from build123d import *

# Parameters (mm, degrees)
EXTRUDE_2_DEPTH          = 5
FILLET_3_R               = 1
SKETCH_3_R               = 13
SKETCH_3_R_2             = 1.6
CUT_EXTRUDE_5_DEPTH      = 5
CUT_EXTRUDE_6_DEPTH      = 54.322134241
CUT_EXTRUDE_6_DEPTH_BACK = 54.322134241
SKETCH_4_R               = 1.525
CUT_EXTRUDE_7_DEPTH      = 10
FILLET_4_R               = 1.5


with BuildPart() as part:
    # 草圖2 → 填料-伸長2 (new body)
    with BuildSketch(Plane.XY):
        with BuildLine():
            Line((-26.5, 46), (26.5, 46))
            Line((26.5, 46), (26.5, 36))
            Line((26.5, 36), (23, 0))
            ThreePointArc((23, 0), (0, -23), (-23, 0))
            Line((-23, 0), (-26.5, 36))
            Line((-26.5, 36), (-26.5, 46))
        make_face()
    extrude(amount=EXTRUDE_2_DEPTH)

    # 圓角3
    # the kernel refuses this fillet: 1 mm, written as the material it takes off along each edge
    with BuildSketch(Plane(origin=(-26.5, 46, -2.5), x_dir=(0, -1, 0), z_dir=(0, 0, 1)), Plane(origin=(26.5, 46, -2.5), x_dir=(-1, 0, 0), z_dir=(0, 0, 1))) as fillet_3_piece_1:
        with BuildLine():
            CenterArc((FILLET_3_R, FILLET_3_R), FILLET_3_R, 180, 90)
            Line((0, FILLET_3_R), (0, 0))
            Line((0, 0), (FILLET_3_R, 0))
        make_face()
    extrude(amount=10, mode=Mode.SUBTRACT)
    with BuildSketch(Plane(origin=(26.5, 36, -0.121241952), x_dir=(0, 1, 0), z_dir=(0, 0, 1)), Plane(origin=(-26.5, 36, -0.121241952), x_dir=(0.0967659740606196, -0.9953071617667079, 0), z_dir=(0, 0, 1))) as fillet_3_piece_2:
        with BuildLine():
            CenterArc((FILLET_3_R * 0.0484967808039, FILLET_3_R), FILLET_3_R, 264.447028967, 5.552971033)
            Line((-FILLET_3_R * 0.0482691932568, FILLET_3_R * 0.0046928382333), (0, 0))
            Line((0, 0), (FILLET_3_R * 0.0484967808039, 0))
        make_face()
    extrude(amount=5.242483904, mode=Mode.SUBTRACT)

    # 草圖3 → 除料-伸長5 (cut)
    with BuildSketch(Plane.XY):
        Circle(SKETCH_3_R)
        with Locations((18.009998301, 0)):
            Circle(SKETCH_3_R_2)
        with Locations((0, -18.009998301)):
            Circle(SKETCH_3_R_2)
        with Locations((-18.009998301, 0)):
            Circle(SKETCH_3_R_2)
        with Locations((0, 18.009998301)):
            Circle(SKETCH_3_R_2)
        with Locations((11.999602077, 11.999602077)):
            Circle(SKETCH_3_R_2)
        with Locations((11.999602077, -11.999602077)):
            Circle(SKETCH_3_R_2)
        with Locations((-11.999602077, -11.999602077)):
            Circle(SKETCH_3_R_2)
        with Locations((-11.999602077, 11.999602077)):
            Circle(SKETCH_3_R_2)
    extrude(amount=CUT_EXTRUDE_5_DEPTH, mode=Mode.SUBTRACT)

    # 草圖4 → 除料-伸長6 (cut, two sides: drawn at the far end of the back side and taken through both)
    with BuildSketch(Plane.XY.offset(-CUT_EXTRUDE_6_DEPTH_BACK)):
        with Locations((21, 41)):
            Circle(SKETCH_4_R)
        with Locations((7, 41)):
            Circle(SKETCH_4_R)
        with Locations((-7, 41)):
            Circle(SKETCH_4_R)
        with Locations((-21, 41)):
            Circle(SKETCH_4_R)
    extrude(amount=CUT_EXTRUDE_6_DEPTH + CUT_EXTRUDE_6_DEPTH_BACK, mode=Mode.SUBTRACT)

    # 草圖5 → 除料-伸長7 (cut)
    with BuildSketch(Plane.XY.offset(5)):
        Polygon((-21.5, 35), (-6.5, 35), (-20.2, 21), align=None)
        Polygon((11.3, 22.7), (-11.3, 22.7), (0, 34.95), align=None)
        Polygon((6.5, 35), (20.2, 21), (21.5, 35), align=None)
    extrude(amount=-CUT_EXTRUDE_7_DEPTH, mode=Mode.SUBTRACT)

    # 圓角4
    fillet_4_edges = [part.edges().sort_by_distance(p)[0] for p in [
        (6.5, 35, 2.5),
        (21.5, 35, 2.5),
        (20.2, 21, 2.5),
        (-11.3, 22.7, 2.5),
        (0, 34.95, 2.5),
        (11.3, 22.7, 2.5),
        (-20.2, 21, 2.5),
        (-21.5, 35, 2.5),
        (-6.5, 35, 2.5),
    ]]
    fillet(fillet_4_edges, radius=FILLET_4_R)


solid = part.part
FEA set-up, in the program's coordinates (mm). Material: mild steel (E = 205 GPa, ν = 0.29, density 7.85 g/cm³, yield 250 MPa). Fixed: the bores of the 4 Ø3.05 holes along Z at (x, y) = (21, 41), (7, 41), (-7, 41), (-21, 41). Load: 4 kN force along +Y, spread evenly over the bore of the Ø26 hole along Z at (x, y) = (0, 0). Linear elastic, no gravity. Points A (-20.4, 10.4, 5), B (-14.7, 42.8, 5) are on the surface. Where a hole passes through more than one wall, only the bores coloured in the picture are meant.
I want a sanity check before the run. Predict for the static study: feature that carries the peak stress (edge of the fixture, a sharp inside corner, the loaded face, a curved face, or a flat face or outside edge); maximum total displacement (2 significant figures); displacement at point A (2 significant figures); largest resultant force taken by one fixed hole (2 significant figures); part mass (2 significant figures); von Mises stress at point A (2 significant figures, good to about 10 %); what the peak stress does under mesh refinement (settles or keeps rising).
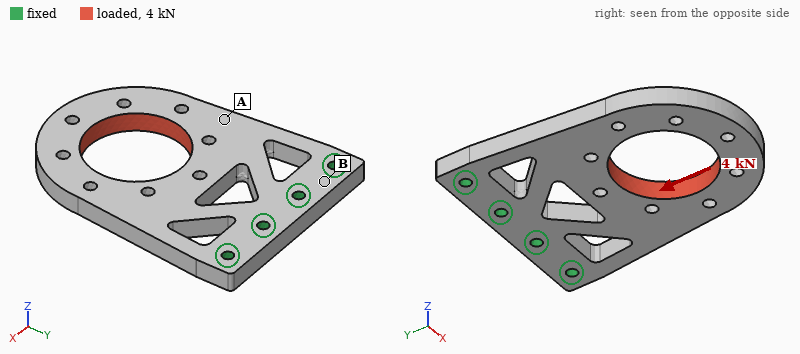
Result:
a sharp inside corner
12 µm
6.2 µm
1.1 kN
86 g
27 MPa
keeps rising
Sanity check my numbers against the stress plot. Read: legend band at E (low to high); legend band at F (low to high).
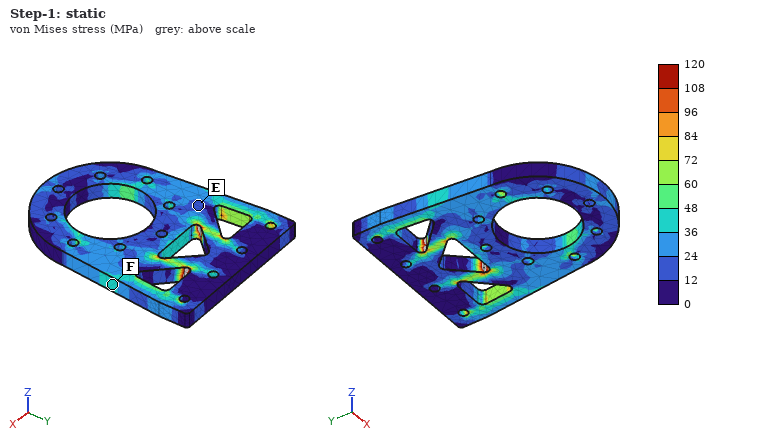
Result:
12 to 24 MPa
36 to 48 MPa
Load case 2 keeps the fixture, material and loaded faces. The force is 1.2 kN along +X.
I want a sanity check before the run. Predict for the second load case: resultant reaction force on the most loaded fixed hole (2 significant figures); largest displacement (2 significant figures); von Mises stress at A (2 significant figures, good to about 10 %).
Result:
1.1 kN
23 µm
14 MPa
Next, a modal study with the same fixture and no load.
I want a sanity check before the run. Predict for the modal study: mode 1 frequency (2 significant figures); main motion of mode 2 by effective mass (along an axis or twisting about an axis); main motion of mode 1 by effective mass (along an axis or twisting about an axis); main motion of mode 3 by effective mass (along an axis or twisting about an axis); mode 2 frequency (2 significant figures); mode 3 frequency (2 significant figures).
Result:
1000 Hz
twisting about Y
along Z
along Z
3100 Hz
5400 Hz
